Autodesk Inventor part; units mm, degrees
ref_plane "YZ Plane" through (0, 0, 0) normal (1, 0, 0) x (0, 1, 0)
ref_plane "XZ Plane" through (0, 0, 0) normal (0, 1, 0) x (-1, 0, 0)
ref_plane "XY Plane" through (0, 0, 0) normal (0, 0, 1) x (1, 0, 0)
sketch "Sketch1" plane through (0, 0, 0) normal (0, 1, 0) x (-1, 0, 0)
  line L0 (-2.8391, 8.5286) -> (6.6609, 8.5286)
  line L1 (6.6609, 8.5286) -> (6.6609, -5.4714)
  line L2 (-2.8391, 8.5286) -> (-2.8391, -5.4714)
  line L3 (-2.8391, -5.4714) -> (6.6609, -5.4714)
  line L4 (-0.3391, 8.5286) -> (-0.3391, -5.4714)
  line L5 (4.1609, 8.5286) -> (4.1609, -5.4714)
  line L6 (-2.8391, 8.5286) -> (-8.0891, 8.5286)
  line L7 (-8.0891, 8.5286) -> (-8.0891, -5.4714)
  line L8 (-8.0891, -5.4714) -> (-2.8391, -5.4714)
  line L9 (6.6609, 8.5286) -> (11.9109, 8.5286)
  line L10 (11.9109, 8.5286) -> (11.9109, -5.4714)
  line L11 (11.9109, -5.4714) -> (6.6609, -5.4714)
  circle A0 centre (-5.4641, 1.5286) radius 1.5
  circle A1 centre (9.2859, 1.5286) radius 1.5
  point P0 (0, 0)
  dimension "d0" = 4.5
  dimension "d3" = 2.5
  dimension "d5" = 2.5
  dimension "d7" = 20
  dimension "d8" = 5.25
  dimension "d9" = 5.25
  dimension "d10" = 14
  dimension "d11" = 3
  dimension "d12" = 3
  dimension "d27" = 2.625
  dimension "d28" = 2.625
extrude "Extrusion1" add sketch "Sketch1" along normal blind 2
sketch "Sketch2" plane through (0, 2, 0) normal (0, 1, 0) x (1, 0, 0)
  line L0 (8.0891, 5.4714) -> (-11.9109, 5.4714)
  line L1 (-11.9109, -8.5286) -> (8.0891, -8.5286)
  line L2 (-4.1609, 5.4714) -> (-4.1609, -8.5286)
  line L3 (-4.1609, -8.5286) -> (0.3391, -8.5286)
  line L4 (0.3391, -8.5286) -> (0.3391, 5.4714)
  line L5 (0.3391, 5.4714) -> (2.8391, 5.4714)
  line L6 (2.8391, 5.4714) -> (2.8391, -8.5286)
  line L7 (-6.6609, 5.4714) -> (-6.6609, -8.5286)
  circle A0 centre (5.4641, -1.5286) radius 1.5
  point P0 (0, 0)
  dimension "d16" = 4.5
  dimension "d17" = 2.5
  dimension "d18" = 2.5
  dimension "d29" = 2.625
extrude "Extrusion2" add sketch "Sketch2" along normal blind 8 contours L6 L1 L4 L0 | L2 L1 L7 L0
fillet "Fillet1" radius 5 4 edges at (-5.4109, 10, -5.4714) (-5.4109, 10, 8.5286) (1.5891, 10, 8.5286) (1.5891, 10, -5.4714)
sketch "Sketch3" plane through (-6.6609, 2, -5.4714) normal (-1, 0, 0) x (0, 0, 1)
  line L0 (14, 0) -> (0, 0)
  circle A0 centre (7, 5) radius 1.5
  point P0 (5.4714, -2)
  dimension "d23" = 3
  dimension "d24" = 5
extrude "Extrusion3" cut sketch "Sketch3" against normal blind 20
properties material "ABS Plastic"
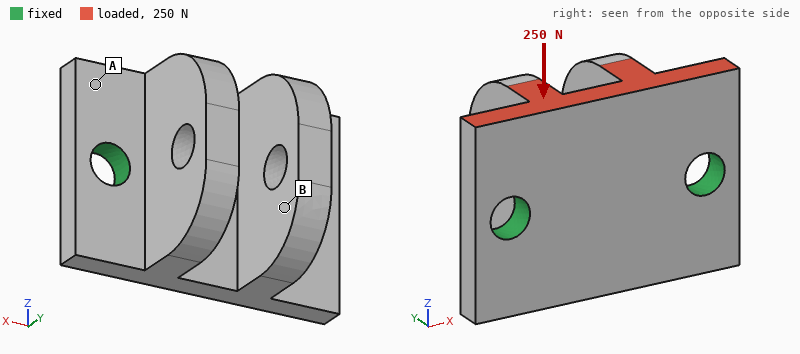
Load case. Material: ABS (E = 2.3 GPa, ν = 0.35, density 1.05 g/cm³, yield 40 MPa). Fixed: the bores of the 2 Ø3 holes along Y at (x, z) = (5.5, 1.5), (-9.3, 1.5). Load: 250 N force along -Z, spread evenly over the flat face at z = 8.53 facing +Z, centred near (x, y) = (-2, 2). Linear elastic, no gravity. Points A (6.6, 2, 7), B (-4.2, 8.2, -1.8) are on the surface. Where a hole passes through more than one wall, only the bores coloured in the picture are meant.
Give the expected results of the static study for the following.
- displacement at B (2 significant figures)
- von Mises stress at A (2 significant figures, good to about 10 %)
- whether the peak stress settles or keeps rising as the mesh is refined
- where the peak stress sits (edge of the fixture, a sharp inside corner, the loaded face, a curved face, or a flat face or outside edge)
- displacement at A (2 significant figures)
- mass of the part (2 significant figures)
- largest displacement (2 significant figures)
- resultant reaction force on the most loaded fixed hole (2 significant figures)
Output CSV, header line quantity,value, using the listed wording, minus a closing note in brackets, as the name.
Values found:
quantity,value
displacement at B,68 µm
von Mises stress at A,5.5 MPa
whether the peak stress settles or keeps rising as the mesh is refined,keeps rising
where the peak stress sits,edge of the fixture
displacement at A,24 µm
mass of the part,1.1 g
largest displacement,79 µm
resultant reaction force on the most loaded fixed hole,130 N
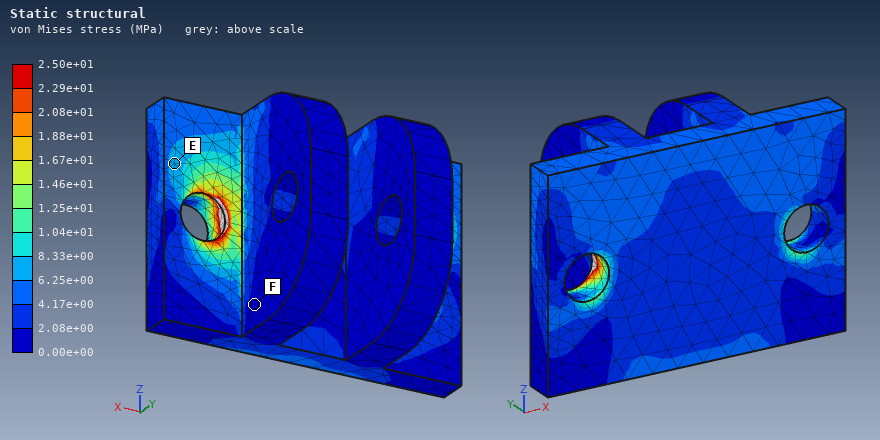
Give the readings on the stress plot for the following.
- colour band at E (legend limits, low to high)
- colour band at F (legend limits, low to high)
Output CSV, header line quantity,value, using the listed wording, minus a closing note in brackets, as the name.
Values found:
quantity,value
colour band at E,6.25e+00 to 8.33e+00 MPa
colour band at F,0.00e+00 to 2.08e+00 MPa
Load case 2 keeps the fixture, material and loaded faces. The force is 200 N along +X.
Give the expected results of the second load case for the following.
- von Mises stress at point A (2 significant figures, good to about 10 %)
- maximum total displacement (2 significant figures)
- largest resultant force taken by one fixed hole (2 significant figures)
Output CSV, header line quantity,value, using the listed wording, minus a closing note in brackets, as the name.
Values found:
quantity,value
von Mises stress at point A,4.4 MPa
maximum total displacement,78 µm
largest resultant force taken by one fixed hole,130 N
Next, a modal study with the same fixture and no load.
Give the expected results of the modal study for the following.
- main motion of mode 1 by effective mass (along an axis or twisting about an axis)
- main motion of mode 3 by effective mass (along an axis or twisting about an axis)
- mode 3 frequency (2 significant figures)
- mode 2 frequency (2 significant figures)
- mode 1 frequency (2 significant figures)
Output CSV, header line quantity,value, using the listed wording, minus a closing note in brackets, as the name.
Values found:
quantity,value
main motion of mode 1 by effective mass,along Z
main motion of mode 3 by effective mass,along X
mode 3 frequency,7900 Hz
mode 2 frequency,5400 Hz
mode 1 frequency,4800 Hz
